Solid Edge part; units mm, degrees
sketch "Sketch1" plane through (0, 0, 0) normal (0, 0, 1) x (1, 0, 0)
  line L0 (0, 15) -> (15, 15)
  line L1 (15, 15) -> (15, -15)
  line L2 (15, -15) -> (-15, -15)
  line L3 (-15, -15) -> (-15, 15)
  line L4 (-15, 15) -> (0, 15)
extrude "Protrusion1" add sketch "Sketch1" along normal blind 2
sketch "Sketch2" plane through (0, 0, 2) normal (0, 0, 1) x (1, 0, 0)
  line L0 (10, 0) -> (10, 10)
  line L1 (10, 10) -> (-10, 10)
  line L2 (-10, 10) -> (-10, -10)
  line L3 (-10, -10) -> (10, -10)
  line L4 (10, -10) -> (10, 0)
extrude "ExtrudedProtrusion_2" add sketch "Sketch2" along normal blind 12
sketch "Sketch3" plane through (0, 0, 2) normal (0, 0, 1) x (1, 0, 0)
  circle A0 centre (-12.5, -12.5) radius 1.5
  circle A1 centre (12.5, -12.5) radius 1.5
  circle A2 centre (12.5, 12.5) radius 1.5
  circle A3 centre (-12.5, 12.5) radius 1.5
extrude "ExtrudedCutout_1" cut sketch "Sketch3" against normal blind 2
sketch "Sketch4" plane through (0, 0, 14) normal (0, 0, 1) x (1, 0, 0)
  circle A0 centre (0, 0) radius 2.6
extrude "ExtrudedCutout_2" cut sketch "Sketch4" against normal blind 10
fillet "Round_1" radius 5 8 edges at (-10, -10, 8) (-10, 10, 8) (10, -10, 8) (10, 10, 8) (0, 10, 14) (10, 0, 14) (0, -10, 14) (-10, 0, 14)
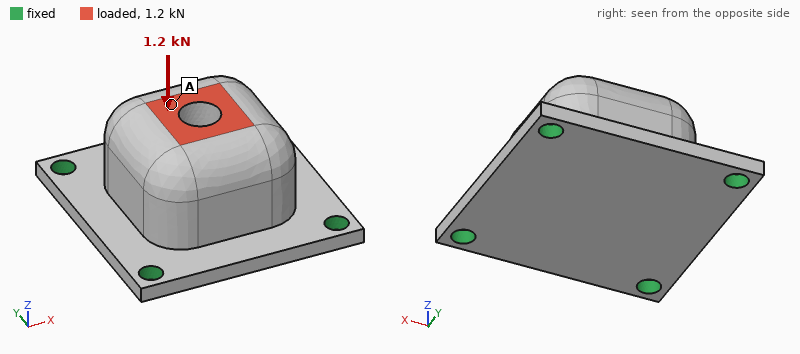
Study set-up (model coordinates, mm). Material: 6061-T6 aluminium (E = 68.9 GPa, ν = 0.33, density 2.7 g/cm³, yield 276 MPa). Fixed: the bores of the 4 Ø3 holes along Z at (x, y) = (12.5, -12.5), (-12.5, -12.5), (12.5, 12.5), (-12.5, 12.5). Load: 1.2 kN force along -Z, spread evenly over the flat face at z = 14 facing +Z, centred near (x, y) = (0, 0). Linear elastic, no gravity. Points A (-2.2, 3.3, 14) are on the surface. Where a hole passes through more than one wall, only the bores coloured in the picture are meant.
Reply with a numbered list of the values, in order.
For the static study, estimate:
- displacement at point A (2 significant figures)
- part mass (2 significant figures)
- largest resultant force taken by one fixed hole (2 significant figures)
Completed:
1. 20 µm
2. 15 g
3. 330 N
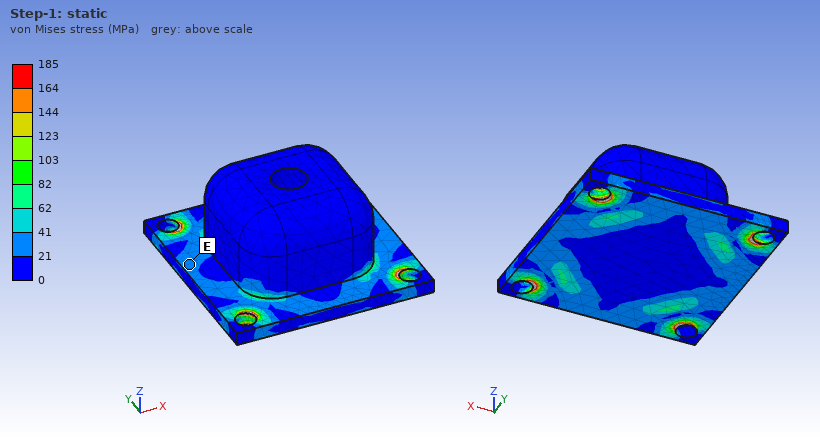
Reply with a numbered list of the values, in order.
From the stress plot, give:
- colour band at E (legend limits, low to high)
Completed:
1. 21 to 41 MPa
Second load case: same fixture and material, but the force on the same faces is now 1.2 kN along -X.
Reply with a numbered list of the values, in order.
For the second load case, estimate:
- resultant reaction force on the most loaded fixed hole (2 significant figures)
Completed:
1. 510 N
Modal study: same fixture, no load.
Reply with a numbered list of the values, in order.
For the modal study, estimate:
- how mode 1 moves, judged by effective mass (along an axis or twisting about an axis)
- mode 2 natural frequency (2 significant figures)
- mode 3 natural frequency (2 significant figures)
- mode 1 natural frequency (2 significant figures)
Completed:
1. along Z
2. 12 kHz
3. 12 kHz
4. 11 kHz
